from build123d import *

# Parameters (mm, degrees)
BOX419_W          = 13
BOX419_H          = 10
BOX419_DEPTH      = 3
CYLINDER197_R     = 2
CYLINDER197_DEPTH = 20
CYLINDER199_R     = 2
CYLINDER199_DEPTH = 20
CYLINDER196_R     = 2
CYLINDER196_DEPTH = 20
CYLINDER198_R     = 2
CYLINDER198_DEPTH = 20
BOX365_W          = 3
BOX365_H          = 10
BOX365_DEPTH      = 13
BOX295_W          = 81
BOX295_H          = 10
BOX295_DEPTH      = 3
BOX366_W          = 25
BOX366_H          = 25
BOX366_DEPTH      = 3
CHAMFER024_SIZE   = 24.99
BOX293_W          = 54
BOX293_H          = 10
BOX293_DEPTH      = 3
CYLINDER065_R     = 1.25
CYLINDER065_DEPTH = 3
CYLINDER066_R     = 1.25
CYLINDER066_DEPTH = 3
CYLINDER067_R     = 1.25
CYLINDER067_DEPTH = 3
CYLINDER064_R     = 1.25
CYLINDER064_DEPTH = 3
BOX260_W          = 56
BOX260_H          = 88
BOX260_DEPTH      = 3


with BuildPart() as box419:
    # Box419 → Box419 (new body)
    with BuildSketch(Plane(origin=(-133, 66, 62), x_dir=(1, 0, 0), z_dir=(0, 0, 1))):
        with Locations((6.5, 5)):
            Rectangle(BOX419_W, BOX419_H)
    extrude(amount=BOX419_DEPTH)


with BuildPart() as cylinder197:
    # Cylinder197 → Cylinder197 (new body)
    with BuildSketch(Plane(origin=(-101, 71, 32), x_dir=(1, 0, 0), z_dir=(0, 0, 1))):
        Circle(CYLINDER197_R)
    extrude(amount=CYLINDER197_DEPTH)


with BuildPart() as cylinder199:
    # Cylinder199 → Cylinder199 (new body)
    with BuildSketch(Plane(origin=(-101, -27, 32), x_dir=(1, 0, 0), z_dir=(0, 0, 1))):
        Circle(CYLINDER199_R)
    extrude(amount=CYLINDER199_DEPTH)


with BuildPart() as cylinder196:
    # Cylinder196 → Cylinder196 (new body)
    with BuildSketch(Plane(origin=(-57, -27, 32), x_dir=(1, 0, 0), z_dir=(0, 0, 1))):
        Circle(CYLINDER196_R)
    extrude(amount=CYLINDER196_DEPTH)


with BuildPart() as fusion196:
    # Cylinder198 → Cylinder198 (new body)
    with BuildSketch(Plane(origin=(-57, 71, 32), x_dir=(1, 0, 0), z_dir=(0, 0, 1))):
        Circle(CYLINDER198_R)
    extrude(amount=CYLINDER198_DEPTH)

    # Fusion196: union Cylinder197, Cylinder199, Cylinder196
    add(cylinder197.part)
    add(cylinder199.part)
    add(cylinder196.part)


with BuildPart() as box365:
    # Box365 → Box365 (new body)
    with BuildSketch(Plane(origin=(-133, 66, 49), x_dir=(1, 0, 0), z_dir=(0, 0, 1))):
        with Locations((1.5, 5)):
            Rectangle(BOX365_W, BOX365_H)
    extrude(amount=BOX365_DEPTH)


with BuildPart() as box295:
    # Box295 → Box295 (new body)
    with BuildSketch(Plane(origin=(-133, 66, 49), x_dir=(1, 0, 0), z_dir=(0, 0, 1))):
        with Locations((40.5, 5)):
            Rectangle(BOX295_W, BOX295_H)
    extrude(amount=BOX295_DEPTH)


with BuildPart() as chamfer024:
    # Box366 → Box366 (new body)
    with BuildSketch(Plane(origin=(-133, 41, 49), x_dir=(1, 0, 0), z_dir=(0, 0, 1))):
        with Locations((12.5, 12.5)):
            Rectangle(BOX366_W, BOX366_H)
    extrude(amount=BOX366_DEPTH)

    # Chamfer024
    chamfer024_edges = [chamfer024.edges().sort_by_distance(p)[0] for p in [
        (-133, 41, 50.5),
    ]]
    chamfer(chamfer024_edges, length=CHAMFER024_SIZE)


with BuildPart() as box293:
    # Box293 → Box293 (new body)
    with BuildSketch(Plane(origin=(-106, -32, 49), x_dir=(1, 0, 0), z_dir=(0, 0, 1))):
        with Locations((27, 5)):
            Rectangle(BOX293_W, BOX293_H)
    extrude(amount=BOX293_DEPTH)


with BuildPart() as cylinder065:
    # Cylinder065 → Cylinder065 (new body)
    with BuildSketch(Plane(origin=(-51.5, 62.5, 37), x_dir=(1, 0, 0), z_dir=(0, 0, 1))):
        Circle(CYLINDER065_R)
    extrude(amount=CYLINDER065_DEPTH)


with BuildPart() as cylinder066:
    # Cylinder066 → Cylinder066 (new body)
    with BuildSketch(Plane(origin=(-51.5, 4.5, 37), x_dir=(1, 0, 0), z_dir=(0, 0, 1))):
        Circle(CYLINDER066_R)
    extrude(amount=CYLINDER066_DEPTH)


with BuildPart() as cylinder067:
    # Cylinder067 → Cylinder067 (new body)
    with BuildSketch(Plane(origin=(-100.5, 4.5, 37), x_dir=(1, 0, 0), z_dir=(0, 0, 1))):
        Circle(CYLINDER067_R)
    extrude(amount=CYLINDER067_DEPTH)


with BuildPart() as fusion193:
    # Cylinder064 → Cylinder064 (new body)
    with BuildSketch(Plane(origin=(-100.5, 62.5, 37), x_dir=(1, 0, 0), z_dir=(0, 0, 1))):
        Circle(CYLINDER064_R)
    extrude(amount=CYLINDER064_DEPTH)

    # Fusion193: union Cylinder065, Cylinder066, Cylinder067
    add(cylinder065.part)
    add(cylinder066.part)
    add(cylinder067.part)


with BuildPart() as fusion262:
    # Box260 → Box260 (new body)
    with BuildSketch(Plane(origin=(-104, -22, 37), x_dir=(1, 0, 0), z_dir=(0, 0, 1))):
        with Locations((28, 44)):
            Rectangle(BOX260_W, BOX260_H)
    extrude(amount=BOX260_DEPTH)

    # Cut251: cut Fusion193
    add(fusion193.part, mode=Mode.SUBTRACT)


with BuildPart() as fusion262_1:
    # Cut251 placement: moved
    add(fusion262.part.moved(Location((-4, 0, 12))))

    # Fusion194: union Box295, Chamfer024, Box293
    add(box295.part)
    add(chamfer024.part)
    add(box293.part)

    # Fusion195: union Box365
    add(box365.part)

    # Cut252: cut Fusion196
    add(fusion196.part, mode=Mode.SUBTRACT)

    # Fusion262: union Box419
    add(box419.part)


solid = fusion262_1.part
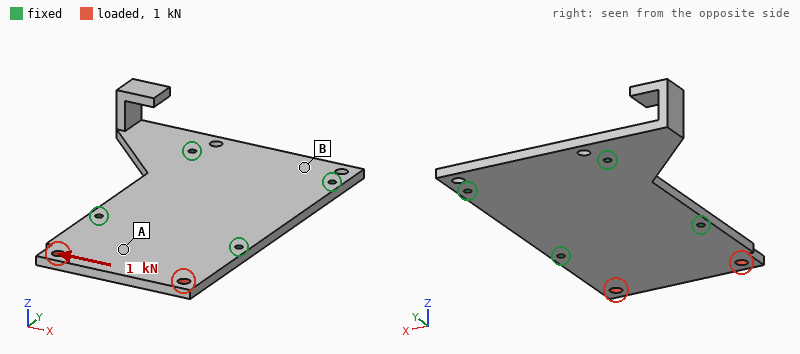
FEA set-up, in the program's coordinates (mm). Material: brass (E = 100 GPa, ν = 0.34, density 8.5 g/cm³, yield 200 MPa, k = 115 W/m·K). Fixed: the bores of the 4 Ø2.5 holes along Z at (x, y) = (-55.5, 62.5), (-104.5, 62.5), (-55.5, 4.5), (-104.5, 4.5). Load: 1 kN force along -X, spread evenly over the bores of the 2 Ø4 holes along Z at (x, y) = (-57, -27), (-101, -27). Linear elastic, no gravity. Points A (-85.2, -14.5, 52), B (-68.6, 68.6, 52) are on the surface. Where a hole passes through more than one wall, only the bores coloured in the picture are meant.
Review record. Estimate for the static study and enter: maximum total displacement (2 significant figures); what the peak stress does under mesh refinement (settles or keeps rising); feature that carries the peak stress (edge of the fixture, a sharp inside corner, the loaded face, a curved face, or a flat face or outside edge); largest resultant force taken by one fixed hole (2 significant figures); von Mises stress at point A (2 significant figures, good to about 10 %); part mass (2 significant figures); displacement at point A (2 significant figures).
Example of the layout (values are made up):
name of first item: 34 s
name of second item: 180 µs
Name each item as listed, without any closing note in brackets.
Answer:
maximum total displacement: 13 µm
what the peak stress does under mesh refinement: keeps rising
feature that carries the peak stress: edge of the fixture
largest resultant force taken by one fixed hole: 780 N
von Mises stress at point A: 14 MPa
part mass: 170 g
displacement at point A: 5.6 µm
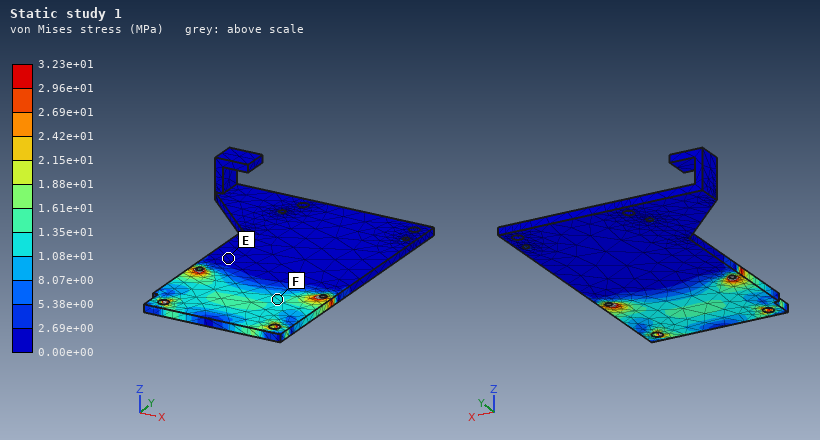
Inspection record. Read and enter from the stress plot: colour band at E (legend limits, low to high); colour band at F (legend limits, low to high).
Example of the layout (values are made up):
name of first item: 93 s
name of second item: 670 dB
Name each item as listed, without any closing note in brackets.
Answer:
colour band at E: 0.00e+00 to 2.69e+00 MPa
colour band at F: 1.08e+01 to 1.35e+01 MPa
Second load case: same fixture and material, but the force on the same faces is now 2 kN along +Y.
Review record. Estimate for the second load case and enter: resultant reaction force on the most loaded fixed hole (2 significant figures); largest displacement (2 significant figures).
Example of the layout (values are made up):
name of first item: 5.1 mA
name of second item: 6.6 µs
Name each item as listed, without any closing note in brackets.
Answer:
resultant reaction force on the most loaded fixed hole: 860 N
largest displacement: 11 µm
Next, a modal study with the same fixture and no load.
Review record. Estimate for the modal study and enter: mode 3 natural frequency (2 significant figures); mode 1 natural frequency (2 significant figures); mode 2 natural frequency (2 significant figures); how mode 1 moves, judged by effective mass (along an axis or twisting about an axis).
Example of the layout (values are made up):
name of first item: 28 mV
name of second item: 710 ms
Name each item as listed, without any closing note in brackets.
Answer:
mode 3 natural frequency: 2300 Hz
mode 1 natural frequency: 1000 Hz
mode 2 natural frequency: 1300 Hz
how mode 1 moves, judged by effective mass: along Z
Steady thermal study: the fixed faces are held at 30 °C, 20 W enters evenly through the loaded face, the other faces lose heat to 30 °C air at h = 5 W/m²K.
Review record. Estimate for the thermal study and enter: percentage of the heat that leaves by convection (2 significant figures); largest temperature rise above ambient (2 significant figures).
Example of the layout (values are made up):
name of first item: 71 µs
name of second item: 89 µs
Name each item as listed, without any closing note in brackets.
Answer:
percentage of the heat that leaves by convection: 3.8 %
largest temperature rise above ambient: 54 K
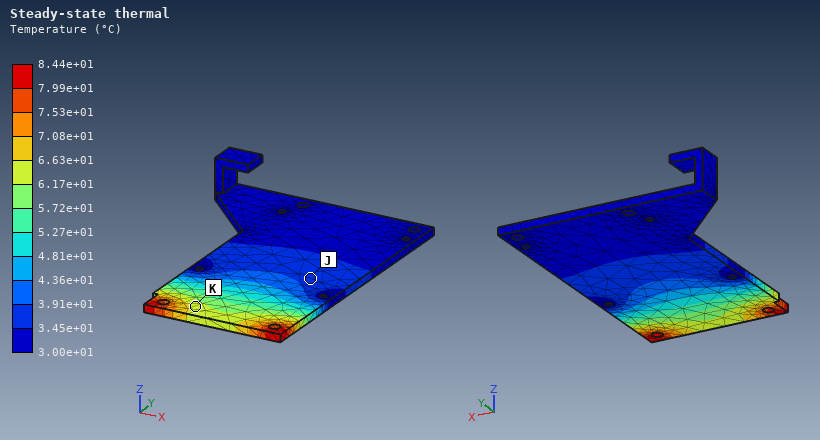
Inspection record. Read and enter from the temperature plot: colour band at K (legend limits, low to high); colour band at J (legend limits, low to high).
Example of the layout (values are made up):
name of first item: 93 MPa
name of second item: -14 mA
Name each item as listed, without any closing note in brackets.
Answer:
colour band at K: 6.17e+01 to 6.63e+01 °C
colour band at J: 3.45e+01 to 3.91e+01 °C
